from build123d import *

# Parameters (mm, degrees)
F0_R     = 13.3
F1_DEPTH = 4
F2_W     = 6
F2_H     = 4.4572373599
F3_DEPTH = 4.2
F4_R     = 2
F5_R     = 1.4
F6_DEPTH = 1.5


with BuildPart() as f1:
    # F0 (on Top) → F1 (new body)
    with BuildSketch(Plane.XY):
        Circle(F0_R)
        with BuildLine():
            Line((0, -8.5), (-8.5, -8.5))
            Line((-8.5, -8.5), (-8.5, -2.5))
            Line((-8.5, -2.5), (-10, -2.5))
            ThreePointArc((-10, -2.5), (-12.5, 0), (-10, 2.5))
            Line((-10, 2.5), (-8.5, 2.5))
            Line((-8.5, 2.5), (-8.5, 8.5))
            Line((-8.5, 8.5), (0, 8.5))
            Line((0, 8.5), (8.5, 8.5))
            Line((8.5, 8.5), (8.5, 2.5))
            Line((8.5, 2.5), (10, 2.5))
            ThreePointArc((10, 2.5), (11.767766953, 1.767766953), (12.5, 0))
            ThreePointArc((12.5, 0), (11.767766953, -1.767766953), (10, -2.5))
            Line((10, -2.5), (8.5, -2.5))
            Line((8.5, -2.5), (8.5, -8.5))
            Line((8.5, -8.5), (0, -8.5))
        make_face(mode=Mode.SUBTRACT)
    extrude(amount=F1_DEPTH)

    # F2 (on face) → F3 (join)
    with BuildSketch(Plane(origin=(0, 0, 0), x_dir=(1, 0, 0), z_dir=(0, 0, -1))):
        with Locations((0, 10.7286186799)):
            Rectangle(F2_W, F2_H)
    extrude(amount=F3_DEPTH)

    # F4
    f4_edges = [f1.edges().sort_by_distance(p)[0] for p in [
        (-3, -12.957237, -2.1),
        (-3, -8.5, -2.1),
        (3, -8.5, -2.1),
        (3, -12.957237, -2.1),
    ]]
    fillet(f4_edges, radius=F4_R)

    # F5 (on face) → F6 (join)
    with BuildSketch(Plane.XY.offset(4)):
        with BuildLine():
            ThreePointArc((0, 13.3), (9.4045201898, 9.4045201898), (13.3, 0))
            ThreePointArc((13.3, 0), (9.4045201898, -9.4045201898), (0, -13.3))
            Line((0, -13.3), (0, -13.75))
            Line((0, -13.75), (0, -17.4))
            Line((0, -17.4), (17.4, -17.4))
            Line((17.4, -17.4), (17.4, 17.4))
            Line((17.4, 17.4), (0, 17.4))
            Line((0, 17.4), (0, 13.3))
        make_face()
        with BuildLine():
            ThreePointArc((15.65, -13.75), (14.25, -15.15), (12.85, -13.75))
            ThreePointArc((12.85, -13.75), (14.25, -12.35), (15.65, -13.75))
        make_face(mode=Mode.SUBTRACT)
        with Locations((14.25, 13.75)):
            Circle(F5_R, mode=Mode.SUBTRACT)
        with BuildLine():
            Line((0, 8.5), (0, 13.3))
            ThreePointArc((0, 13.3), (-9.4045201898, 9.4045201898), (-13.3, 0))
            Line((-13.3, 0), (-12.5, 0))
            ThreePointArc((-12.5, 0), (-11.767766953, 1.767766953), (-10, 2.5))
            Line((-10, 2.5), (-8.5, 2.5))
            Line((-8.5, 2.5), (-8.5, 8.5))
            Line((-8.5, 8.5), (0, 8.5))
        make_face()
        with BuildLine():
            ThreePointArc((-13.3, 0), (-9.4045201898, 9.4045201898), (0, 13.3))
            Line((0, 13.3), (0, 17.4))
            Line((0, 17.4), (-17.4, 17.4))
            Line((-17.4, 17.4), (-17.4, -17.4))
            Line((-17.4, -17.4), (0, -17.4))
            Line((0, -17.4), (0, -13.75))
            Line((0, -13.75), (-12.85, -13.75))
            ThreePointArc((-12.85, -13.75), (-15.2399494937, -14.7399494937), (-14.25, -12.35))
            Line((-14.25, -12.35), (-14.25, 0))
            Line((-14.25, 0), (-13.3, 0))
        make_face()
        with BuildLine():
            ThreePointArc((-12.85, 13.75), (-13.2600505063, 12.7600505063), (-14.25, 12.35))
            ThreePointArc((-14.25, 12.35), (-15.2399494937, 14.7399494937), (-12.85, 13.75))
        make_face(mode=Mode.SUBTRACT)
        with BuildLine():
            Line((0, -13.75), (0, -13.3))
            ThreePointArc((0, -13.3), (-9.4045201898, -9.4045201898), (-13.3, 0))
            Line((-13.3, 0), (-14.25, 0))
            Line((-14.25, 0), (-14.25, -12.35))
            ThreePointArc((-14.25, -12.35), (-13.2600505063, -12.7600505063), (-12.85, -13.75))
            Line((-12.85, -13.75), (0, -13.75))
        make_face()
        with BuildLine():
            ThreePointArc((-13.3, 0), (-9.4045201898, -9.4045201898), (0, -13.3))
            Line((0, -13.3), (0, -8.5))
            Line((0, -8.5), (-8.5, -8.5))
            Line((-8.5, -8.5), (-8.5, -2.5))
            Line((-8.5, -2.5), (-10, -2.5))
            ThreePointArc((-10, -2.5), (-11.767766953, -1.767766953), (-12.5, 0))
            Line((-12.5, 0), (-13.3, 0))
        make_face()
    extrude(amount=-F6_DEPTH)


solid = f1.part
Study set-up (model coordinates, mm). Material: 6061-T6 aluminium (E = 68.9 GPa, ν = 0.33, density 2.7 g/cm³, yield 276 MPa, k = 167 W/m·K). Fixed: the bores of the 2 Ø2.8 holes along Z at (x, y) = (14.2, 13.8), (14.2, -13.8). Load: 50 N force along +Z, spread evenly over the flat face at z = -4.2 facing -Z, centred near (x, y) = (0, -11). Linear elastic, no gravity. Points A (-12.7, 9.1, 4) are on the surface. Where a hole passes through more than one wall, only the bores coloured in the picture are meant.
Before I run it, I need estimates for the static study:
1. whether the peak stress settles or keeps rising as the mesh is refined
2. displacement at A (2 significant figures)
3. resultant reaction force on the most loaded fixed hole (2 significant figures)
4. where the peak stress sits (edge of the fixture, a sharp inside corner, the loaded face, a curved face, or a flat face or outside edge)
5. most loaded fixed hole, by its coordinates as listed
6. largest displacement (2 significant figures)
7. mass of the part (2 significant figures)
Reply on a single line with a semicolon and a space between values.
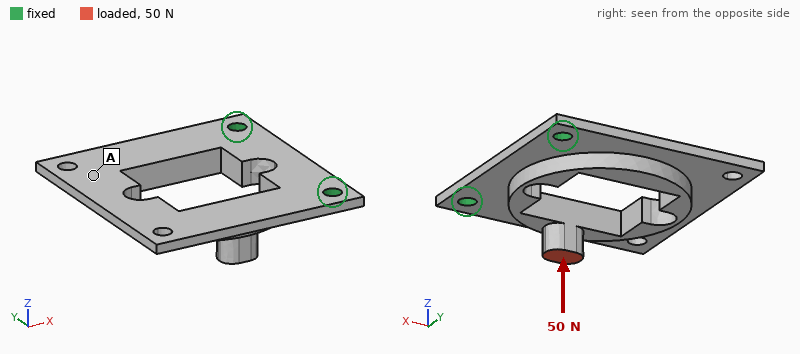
keeps rising; 0.15 mm; 46 N; edge of the fixture; (14.2, -13.8); 0.22 mm; 5.3 g
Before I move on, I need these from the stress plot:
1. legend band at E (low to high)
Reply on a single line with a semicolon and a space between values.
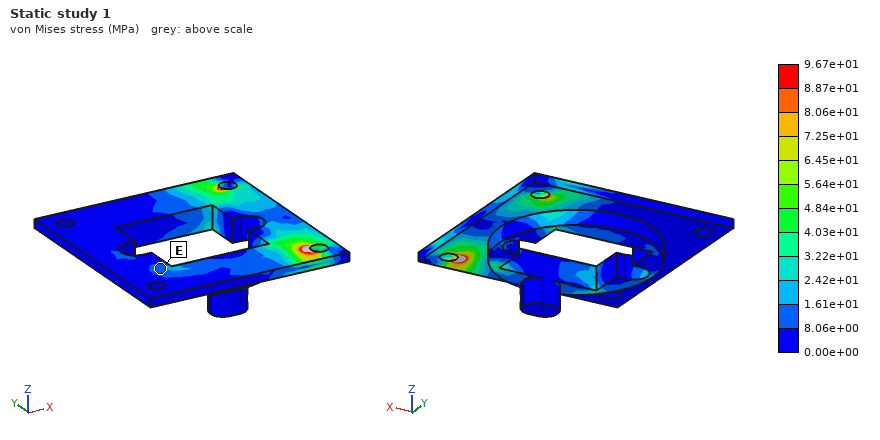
8.06e+00 to 1.61e+01 MPa
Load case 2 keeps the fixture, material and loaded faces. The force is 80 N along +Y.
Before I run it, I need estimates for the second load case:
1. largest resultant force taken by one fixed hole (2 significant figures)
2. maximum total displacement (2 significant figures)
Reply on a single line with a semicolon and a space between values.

59 N; 55 µm
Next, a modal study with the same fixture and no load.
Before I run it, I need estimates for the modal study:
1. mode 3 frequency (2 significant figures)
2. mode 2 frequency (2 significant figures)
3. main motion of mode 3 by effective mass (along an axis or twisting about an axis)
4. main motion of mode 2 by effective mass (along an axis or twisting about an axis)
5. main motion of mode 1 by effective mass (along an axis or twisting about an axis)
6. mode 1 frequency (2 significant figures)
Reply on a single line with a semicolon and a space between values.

8200 Hz; 3900 Hz; along Y; twisting about X; along Z; 1300 Hz
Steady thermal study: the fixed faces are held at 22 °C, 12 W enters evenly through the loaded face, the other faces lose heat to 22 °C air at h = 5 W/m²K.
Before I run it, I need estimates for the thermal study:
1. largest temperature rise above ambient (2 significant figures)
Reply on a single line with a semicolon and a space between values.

57 K
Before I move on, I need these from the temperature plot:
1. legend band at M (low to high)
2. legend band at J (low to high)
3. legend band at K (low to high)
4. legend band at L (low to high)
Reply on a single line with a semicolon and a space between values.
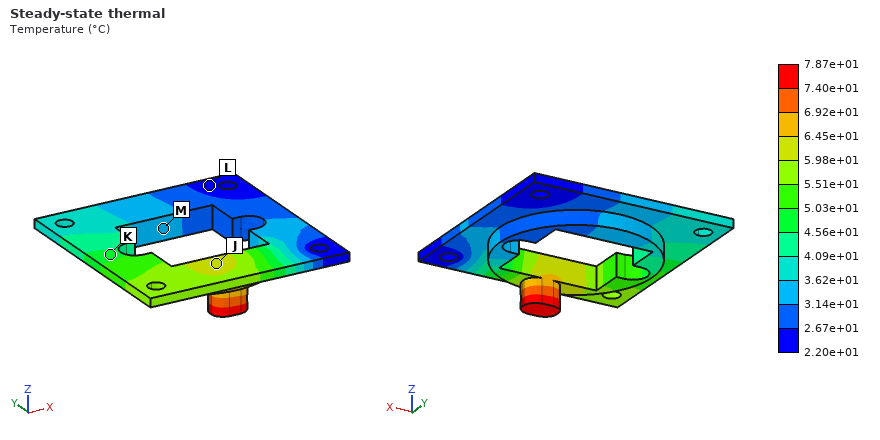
3.14e+01 to 3.62e+01 °C; 5.98e+01 to 6.45e+01 °C; 4.56e+01 to 5.03e+01 °C; 2.20e+01 to 2.67e+01 °C
